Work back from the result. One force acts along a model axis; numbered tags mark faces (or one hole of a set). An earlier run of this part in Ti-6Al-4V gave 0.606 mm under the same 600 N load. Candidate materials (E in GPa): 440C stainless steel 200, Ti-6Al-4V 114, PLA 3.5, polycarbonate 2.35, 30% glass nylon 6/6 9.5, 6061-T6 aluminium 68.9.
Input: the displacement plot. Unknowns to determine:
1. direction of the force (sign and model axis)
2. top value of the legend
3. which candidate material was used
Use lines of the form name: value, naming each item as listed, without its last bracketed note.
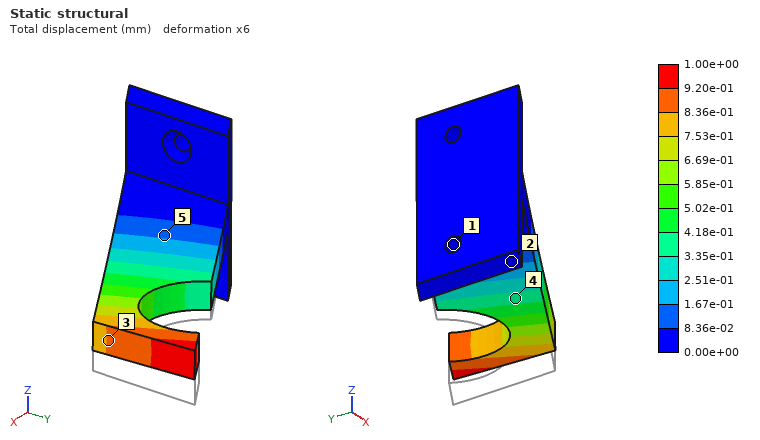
direction of the force: +Z
top value of the legend: 1.00e+00 mm
which candidate material was used: 6061-T6 aluminium
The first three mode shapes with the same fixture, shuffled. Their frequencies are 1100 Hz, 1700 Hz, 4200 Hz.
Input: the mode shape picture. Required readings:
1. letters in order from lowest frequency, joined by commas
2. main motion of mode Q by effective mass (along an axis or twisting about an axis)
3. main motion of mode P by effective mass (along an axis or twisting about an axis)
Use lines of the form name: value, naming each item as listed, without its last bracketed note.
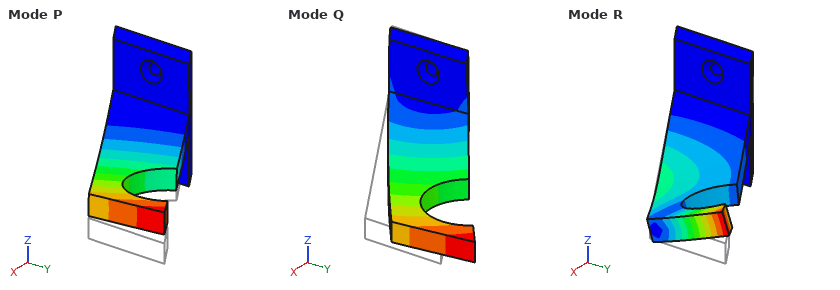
letters in order from lowest frequency, joined by commas: P, Q, R
main motion of mode Q by effective mass: along Y
main motion of mode P by effective mass: along Z
